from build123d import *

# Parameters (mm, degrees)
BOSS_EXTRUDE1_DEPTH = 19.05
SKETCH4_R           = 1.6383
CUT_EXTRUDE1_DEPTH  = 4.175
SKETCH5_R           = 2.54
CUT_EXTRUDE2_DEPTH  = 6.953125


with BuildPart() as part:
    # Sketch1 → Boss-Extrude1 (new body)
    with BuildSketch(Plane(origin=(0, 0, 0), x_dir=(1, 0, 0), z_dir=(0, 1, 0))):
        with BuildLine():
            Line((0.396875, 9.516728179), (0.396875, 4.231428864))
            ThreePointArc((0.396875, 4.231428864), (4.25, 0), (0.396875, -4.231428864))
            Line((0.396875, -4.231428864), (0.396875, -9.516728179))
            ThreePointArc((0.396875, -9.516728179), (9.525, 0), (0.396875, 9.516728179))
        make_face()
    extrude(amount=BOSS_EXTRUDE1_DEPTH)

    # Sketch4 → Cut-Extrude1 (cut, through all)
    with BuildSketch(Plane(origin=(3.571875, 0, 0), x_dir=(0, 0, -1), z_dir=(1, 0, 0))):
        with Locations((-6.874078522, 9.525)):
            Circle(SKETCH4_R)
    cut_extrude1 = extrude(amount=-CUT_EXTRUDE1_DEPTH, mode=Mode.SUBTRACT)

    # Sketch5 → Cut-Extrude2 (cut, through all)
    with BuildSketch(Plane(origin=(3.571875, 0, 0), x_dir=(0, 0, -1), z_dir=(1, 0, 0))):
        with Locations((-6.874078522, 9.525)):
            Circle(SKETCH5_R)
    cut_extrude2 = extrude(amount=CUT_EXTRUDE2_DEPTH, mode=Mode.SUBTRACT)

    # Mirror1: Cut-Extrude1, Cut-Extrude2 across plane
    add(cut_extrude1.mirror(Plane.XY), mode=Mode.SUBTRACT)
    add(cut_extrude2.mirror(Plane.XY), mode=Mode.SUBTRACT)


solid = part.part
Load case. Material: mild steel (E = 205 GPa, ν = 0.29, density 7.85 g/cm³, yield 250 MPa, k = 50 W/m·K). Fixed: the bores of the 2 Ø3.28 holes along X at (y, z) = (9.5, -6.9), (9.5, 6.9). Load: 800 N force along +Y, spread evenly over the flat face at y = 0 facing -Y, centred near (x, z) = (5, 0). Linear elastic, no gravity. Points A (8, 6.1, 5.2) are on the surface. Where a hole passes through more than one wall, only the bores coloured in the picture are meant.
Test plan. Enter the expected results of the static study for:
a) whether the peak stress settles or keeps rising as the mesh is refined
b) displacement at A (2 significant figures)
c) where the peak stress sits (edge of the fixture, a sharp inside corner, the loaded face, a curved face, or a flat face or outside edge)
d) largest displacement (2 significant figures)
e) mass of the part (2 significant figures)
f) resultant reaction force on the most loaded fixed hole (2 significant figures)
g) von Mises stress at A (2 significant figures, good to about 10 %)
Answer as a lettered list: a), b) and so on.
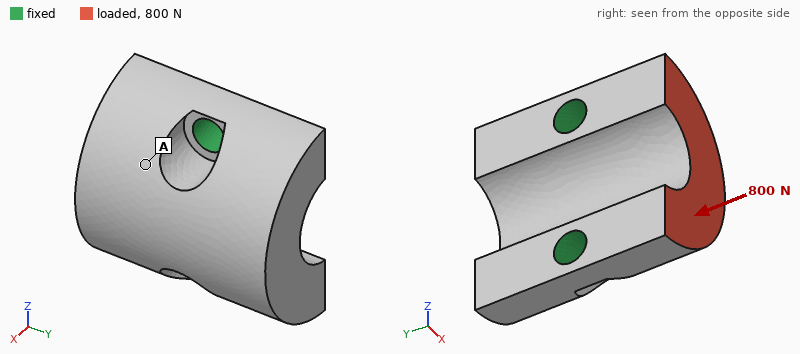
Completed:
a) keeps rising
b) 2.2 µm
c) edge of the fixture
d) 3.8 µm
e) 15 g
f) 400 N
g) 10 MPa
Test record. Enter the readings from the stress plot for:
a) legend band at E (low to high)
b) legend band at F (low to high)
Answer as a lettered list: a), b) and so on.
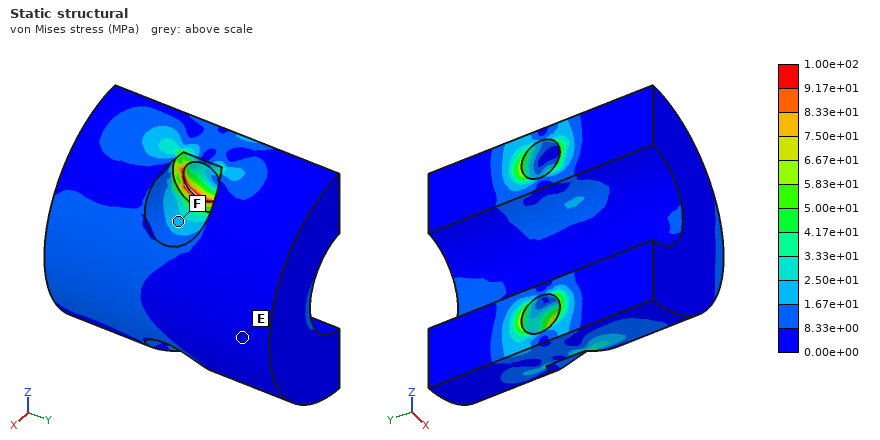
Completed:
a) 0.00e+00 to 8.33e+00 MPa
b) 1.67e+01 to 2.50e+01 MPa
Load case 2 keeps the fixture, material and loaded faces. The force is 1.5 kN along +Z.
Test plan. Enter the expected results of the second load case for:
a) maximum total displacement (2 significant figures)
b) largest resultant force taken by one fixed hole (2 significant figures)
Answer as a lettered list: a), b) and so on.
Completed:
a) 7.7 µm
b) 1.1 kN
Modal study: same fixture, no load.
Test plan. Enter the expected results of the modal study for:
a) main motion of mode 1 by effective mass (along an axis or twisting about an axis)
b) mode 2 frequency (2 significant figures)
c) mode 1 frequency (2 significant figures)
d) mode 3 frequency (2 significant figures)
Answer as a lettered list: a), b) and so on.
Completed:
a) along Y
b) 43 kHz
c) 19 kHz
d) 44 kHz
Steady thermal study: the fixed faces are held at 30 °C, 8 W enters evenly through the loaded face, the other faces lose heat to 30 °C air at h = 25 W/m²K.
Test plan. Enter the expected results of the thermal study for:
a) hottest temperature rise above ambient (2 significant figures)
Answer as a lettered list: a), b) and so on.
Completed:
a) 18 K
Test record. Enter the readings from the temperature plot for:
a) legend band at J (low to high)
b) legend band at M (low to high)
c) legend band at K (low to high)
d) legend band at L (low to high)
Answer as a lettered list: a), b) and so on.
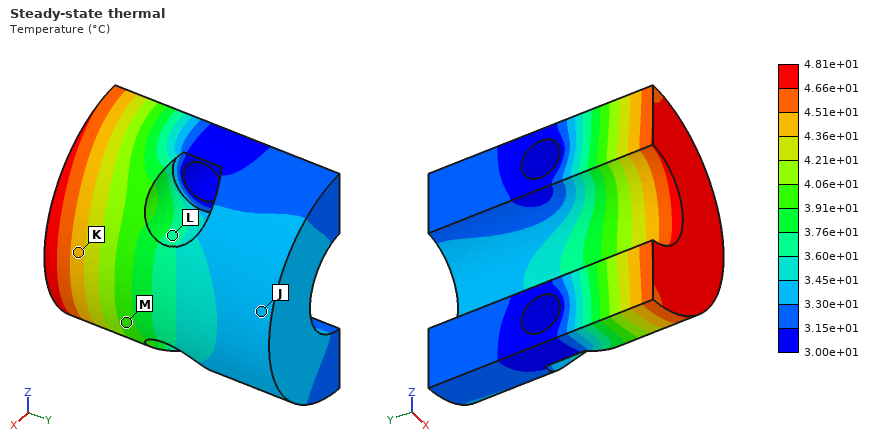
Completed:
a) 3.30e+01 to 3.45e+01 °C
b) 3.91e+01 to 4.06e+01 °C
c) 4.36e+01 to 4.51e+01 °C
d) 3.60e+01 to 3.76e+01 °C
